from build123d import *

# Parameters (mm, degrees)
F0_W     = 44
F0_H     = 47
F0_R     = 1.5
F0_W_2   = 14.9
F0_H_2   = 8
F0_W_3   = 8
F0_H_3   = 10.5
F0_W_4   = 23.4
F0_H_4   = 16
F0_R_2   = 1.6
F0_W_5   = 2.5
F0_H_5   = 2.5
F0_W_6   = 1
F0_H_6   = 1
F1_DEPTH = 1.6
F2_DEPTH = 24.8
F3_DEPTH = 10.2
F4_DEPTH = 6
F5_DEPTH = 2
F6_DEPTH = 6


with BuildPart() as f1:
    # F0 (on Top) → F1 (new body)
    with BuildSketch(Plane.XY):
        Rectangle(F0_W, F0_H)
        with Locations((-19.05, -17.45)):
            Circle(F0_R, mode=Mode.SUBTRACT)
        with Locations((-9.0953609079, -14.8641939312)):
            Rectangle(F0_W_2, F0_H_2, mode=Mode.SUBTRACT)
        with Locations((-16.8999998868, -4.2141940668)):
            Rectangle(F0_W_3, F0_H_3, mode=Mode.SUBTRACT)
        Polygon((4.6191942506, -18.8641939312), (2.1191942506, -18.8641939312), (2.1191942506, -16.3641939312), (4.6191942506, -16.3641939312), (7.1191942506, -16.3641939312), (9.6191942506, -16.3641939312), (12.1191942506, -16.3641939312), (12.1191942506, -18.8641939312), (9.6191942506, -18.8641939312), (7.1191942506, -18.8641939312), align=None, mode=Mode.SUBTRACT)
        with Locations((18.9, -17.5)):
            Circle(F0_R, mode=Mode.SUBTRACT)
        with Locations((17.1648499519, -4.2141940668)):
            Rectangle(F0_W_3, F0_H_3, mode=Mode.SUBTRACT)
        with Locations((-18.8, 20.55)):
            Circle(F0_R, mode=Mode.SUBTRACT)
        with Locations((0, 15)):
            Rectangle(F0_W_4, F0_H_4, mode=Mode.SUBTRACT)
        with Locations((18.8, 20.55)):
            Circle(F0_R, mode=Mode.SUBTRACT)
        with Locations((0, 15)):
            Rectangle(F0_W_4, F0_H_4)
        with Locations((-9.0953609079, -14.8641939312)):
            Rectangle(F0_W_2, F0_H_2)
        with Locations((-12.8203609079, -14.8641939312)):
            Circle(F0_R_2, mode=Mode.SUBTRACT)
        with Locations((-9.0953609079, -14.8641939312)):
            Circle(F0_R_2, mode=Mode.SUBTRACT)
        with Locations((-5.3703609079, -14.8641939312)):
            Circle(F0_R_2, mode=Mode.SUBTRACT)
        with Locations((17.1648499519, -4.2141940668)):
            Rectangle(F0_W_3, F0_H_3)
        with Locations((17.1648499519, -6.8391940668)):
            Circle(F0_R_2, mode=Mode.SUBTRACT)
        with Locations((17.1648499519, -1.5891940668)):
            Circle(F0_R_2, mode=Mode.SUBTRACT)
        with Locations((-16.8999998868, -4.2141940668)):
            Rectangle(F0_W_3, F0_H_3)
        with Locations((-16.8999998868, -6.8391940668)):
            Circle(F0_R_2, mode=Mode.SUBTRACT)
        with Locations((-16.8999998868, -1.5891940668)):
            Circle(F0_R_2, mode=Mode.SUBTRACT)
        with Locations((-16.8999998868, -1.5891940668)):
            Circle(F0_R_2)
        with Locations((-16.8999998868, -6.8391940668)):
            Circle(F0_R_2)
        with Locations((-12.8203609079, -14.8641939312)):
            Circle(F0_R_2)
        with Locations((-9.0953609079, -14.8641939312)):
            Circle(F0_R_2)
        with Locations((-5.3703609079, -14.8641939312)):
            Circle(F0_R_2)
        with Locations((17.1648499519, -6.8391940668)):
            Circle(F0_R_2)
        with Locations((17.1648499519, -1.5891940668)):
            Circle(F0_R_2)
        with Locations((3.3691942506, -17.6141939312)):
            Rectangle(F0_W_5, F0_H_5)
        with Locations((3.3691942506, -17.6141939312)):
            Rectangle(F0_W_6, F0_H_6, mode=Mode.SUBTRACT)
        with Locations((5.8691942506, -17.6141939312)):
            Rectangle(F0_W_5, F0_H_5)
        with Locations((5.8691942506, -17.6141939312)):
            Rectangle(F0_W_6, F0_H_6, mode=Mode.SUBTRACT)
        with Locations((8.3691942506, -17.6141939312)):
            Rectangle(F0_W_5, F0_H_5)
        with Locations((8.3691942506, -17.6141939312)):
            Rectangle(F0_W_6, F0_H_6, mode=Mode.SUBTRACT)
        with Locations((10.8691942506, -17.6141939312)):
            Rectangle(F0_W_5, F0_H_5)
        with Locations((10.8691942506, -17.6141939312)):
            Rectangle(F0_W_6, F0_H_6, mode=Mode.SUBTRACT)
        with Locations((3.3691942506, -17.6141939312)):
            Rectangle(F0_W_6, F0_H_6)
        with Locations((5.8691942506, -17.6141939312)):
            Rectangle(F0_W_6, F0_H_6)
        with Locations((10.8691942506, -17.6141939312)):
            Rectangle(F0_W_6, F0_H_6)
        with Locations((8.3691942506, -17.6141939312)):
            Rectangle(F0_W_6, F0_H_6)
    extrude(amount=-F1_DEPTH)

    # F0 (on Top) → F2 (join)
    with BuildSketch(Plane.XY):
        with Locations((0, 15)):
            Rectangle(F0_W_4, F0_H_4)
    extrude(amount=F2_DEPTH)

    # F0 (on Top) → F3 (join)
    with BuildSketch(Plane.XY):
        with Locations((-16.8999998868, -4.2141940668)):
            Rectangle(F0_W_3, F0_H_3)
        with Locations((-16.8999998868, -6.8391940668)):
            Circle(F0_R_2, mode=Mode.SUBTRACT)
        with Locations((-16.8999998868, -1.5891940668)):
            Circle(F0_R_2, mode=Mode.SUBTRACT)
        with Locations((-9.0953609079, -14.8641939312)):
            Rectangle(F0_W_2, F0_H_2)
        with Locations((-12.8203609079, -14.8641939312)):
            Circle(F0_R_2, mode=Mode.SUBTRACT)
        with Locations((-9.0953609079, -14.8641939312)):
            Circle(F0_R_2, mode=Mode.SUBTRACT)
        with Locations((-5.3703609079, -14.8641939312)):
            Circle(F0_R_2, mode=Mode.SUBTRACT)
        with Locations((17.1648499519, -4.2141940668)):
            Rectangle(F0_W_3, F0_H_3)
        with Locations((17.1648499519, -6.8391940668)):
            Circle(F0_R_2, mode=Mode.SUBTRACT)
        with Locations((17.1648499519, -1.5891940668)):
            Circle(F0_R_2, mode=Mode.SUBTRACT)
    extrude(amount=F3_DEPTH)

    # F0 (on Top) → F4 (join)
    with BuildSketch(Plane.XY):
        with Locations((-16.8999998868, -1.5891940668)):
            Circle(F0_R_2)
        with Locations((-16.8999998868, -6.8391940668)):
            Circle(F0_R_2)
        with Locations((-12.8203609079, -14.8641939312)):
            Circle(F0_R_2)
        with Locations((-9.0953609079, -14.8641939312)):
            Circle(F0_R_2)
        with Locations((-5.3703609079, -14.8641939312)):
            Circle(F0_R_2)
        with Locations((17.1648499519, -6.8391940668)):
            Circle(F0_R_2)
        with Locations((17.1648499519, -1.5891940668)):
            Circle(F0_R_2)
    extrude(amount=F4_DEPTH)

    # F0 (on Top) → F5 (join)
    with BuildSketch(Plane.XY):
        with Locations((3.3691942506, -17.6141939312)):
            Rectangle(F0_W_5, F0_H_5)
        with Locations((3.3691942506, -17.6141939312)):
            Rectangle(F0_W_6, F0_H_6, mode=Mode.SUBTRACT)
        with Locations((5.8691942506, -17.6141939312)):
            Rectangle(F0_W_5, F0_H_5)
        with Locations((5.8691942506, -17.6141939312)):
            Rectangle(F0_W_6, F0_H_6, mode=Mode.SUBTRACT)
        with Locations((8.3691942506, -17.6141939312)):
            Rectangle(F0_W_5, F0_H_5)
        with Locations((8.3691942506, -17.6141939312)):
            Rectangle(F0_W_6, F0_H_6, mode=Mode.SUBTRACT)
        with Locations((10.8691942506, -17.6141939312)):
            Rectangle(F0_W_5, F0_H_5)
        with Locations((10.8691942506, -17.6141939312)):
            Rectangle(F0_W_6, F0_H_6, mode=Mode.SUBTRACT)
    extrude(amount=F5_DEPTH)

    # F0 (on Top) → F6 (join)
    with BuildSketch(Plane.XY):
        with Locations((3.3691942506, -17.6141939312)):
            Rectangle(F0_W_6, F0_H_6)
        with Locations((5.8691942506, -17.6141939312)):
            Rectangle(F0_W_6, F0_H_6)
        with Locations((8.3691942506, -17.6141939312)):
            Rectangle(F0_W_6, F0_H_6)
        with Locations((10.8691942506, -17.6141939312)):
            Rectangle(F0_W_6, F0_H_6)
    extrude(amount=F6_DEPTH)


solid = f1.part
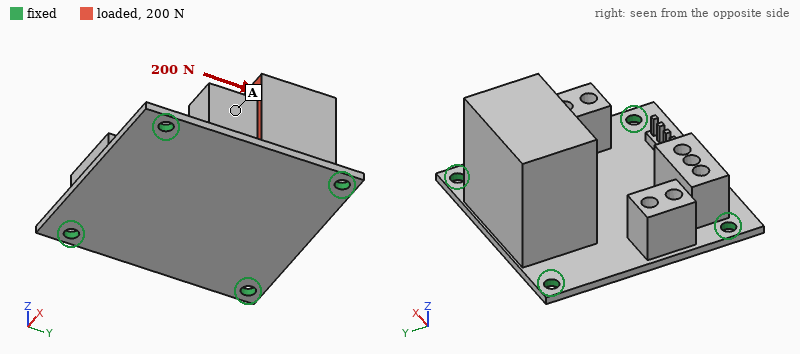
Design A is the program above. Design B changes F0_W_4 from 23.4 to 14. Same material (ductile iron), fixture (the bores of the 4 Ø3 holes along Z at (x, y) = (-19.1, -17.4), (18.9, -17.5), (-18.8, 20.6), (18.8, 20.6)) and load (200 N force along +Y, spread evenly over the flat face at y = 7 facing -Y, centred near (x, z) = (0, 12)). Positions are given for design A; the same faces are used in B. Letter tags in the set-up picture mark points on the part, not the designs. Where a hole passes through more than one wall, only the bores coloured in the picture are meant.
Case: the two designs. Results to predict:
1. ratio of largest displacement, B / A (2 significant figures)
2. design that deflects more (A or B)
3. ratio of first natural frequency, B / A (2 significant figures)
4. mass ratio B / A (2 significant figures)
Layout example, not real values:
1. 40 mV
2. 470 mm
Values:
1. 1.5
2. B
3. 1.1
4. 0.76
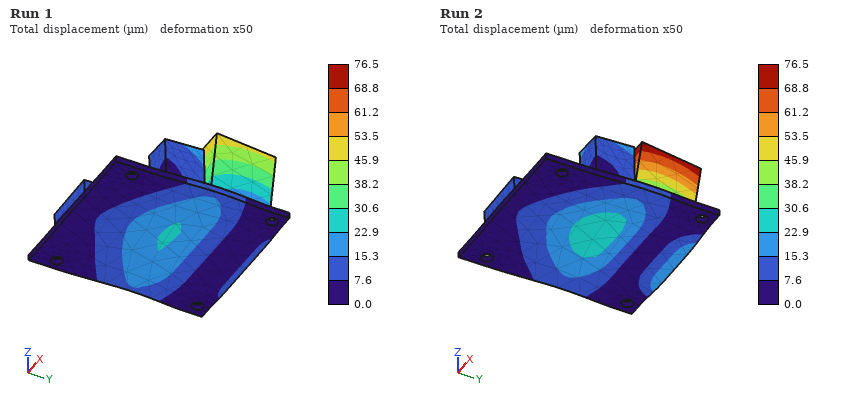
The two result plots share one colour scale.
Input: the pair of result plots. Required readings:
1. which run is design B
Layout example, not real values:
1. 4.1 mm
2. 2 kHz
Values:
1. Run 2
